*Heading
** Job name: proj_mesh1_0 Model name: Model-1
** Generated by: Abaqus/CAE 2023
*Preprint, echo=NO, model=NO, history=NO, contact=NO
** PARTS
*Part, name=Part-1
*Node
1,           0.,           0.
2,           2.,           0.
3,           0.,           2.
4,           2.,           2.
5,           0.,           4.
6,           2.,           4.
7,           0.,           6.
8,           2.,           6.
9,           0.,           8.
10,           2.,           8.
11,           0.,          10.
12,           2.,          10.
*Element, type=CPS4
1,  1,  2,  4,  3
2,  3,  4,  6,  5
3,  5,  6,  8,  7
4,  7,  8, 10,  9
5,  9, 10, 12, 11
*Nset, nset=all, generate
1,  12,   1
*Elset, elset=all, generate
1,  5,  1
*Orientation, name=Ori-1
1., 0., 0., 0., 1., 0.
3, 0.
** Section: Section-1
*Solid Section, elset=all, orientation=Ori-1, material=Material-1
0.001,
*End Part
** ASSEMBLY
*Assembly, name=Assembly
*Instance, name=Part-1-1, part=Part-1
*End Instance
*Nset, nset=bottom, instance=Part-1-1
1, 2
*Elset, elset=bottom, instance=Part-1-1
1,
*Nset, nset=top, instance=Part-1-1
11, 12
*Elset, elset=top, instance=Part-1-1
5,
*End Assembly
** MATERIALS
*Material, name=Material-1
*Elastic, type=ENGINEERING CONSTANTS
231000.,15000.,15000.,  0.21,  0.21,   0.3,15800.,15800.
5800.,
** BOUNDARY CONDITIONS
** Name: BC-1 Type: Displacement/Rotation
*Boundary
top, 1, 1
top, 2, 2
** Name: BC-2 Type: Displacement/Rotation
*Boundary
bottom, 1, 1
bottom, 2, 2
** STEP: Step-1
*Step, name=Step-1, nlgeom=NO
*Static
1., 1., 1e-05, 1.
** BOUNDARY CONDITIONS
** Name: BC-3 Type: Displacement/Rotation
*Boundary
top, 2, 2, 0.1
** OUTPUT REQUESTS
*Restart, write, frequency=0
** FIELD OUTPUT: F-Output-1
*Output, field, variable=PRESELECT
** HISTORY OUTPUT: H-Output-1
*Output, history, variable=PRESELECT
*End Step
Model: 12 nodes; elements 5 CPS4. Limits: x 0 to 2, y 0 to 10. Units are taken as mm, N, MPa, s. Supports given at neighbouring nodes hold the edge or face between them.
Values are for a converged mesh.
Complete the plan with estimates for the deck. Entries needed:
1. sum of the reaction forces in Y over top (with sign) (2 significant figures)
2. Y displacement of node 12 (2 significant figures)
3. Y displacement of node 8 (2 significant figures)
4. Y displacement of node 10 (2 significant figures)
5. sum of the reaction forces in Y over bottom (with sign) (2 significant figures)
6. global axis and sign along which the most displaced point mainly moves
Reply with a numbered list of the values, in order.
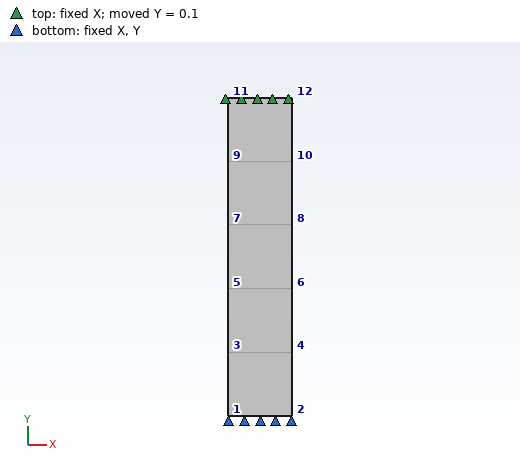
1. 0.30 N
2. 0.10 mm
3. 0.060 mm
4. 0.080 mm
5. -0.30 N
6. +Y
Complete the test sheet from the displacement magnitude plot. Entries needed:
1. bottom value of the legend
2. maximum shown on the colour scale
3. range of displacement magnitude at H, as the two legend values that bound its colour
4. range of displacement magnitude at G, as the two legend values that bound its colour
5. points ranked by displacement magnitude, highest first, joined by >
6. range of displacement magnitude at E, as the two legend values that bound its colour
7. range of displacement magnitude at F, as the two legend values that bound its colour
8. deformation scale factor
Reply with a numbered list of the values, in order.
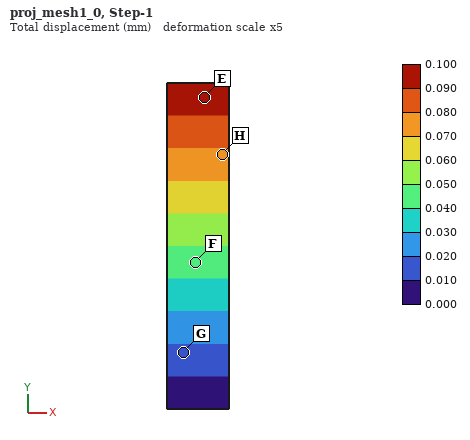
1. 0.000 mm
2. 0.100 mm
3. 0.070 to 0.080 mm
4. 0.010 to 0.020 mm
5. E > H > F > G
6. 0.090 to 0.100 mm
7. 0.040 to 0.050 mm
8. 5
